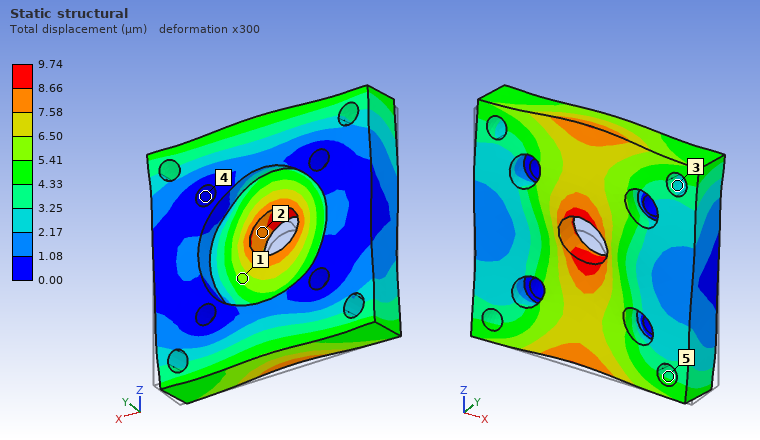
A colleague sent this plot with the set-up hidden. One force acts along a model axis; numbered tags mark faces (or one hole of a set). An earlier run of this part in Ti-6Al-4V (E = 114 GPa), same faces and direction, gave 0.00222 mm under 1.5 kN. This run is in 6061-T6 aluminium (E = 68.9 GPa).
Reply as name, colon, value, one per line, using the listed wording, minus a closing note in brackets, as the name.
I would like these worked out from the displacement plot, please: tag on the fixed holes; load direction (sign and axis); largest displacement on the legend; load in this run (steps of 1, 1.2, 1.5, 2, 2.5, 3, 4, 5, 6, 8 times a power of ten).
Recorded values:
tag on the fixed holes: 4
load direction: +Z
largest displacement on the legend: 9.74 µm
load in this run: 4 kN
